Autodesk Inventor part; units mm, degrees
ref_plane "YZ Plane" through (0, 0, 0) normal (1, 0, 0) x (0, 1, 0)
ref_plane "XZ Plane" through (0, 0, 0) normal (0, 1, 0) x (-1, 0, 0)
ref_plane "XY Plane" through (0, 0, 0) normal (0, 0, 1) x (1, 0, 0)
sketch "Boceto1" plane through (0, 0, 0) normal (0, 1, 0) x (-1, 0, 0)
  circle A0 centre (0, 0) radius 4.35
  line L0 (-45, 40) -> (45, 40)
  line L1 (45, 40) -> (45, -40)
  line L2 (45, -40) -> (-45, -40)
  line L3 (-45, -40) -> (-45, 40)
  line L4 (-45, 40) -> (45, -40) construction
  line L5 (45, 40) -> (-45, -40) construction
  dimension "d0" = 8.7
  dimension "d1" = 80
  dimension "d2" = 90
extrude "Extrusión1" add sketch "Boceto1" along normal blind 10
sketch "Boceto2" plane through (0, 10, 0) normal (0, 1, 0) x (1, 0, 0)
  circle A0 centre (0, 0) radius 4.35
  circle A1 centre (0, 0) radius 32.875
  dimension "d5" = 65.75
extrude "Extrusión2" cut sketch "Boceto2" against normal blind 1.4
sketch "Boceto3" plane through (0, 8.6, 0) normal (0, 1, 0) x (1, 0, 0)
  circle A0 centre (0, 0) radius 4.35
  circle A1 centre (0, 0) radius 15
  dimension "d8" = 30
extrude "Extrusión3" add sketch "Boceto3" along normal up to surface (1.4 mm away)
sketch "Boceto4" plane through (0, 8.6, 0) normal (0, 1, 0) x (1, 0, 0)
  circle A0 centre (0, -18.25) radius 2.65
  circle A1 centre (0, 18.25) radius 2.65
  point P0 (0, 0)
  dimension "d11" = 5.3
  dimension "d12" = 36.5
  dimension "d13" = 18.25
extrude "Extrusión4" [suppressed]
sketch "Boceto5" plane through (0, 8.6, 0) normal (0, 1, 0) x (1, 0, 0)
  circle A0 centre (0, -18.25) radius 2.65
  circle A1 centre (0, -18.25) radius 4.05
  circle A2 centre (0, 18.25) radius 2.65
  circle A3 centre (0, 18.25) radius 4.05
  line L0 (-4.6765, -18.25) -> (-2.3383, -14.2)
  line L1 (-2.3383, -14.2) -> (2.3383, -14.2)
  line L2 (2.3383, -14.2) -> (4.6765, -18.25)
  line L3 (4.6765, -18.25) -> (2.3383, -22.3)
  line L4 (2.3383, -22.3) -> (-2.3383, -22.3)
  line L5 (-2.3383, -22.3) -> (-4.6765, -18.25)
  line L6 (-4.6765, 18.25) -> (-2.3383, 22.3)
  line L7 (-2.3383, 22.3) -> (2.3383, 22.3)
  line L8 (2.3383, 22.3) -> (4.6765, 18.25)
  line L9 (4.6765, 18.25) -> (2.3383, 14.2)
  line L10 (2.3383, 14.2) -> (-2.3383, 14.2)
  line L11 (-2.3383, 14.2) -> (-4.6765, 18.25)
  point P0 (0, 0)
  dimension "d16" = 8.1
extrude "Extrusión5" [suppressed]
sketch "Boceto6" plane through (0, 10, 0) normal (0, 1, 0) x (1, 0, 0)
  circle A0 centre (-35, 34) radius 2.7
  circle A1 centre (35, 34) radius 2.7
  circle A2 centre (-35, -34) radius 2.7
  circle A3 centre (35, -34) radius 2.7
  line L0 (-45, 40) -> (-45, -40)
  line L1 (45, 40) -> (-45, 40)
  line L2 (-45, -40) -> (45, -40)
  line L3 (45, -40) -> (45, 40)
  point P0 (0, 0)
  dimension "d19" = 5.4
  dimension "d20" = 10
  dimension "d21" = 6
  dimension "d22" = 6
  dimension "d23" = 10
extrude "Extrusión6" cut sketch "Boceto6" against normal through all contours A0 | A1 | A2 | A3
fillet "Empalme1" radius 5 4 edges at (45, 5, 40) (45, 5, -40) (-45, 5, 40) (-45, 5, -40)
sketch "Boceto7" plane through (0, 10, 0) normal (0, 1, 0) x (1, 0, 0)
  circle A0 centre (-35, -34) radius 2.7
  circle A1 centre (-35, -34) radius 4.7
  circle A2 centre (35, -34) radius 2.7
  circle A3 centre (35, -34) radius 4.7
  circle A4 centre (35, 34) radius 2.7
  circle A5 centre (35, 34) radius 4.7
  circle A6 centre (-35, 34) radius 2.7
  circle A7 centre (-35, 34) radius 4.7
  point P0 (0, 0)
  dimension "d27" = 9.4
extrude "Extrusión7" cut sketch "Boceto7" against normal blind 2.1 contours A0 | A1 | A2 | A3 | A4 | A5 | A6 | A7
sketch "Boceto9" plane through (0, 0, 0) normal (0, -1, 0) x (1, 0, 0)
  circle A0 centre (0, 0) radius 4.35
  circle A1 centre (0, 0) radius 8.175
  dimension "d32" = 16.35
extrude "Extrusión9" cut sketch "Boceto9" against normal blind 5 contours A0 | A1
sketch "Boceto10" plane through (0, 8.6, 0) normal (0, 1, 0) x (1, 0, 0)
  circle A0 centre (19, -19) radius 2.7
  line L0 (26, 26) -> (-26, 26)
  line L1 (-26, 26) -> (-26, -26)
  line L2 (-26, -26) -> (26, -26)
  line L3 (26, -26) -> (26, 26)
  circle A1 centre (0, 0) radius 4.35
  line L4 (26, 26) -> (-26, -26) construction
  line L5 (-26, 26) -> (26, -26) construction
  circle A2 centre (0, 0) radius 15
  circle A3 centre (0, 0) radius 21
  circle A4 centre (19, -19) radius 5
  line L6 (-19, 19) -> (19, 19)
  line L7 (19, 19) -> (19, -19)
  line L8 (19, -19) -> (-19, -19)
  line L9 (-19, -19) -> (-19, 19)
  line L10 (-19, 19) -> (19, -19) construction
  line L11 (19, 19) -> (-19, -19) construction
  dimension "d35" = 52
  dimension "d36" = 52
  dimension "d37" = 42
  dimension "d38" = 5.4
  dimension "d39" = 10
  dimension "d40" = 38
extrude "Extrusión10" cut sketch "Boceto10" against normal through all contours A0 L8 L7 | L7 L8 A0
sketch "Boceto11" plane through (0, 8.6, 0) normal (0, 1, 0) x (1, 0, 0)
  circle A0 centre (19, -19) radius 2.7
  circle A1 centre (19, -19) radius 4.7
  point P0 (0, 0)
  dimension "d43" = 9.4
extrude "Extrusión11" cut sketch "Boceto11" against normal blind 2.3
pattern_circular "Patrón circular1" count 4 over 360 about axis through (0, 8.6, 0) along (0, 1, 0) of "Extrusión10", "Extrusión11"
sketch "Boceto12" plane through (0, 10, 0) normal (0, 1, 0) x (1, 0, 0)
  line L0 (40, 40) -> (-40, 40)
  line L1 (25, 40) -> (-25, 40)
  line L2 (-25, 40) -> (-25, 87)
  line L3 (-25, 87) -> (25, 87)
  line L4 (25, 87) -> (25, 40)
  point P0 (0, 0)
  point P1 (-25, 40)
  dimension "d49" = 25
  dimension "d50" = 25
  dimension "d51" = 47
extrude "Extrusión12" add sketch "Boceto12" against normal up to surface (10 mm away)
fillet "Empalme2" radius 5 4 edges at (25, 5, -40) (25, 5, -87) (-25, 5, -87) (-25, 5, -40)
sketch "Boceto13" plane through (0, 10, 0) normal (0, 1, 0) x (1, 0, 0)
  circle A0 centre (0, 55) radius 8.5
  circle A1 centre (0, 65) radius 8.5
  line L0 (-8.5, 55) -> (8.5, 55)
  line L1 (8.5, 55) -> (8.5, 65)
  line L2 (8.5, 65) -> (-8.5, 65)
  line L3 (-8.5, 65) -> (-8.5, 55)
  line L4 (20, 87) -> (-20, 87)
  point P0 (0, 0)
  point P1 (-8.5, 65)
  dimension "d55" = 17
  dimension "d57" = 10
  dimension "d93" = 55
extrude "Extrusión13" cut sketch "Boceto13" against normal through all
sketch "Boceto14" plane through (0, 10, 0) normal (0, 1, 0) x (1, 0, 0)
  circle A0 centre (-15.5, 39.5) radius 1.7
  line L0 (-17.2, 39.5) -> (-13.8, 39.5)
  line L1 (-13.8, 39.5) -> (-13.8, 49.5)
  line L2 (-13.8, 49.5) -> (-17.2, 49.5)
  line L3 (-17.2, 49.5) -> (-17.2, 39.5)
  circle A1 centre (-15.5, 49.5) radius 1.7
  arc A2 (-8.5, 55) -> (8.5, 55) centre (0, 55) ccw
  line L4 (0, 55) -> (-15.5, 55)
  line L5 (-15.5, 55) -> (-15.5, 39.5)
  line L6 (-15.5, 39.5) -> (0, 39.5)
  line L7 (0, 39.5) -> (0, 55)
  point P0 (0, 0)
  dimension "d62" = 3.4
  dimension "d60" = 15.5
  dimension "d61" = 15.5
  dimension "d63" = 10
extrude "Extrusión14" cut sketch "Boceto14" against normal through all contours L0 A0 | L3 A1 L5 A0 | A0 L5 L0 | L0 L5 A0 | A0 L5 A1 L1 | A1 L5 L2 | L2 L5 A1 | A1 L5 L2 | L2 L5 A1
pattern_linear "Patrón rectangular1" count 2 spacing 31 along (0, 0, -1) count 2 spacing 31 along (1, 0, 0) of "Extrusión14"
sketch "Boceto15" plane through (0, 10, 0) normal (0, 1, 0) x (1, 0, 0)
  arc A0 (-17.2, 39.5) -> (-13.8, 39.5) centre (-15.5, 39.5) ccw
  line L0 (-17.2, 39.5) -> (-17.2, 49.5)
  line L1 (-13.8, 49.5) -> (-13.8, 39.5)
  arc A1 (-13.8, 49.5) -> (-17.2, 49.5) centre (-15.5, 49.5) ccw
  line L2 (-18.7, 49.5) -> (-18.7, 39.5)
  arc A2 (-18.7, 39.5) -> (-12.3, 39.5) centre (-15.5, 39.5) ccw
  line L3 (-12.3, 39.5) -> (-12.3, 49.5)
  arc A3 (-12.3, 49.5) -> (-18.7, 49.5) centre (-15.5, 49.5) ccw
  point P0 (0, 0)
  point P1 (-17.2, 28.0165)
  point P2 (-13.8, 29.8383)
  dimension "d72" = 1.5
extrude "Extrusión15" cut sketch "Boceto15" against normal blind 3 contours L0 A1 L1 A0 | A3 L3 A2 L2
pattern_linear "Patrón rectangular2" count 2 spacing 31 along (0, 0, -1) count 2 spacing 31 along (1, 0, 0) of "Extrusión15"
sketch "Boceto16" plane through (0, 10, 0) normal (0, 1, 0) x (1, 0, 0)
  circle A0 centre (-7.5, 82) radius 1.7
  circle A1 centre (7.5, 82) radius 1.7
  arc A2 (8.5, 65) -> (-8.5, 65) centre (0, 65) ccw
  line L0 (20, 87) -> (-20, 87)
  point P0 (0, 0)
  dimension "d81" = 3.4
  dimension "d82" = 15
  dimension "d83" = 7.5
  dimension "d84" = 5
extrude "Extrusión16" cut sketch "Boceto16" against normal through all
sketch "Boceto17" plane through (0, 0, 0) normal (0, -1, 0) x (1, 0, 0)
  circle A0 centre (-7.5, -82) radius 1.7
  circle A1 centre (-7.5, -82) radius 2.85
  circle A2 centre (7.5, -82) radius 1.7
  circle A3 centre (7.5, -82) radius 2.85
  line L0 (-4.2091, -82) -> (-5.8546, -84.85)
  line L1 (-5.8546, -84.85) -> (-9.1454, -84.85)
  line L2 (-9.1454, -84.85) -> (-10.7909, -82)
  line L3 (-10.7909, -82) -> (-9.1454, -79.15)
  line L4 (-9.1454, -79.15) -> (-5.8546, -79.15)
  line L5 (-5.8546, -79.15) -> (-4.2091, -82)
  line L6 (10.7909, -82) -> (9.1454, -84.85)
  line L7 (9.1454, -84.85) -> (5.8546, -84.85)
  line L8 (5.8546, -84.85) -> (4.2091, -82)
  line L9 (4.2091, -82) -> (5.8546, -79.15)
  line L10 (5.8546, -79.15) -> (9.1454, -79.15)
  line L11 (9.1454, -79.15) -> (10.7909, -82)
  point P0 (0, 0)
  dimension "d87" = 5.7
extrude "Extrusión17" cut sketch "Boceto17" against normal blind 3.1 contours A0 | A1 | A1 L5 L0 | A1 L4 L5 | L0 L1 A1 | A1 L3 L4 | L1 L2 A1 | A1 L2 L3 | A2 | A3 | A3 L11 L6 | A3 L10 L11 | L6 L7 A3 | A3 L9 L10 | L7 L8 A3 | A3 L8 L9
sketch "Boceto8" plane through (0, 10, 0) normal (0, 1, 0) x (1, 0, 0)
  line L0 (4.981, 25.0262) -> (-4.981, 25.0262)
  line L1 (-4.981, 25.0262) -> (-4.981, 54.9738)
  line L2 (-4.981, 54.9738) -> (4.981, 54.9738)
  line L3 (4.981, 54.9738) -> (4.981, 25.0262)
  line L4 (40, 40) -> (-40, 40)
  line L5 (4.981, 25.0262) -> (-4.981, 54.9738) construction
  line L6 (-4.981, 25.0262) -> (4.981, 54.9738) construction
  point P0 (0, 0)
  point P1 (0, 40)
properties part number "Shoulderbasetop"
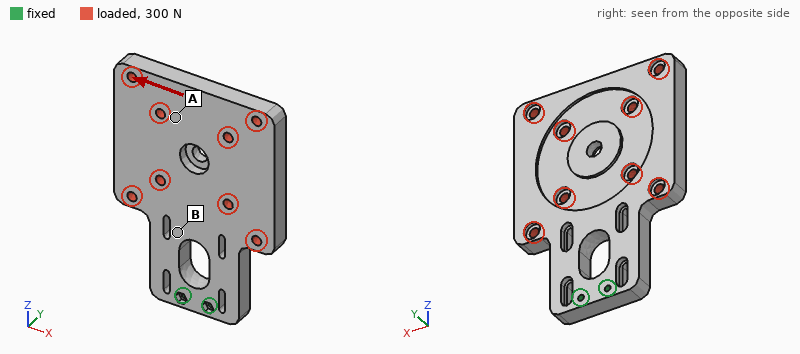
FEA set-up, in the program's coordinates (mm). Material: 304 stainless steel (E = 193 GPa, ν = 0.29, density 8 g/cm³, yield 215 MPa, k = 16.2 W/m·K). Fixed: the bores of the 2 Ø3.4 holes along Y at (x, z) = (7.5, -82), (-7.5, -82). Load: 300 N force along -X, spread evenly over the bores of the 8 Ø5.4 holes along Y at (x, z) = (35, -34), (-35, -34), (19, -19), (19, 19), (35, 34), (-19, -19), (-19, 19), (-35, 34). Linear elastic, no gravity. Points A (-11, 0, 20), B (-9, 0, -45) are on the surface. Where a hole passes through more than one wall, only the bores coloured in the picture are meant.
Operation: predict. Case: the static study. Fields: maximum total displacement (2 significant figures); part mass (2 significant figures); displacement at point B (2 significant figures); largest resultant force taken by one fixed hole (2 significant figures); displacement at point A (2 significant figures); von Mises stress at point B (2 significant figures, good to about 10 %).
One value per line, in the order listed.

31 µm
650 g
9.6 µm
1.3 kN
25 µm
5.4 MPa
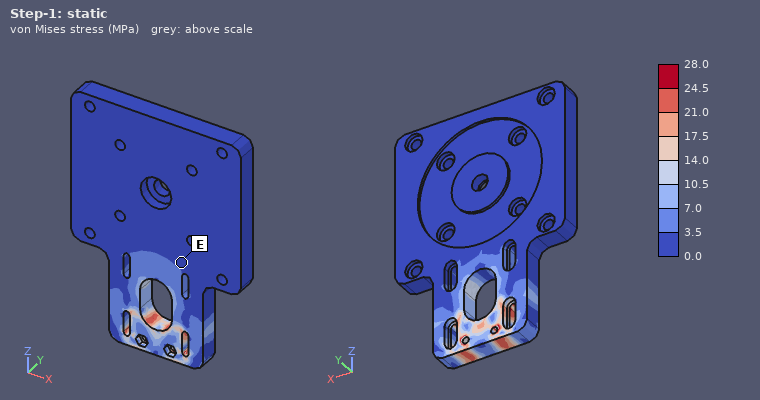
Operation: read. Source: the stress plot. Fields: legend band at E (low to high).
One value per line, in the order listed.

0.0 to 3.5 MPa
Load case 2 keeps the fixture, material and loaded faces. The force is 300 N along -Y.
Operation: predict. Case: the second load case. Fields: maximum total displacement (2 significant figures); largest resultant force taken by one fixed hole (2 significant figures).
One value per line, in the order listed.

0.25 mm
170 N
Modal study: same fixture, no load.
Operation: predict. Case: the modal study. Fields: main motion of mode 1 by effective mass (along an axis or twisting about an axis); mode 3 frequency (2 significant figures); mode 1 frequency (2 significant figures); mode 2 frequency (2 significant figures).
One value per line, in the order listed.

along Y
810 Hz
290 Hz
780 Hz
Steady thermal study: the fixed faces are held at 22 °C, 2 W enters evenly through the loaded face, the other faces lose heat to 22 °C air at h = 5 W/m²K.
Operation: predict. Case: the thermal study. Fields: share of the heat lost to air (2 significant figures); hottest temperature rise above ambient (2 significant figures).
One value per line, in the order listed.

58 %
13 K
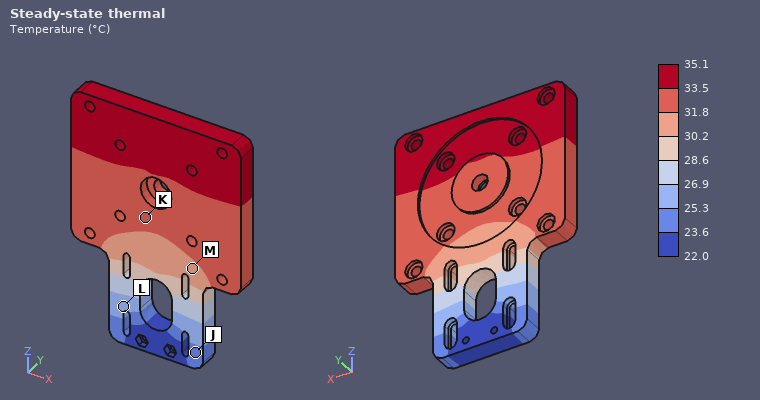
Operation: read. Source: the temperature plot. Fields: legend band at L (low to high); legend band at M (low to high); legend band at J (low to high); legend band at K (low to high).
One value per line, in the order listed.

25.3 to 26.9 °C
30.2 to 31.8 °C
23.6 to 25.3 °C
31.8 to 33.5 °C
